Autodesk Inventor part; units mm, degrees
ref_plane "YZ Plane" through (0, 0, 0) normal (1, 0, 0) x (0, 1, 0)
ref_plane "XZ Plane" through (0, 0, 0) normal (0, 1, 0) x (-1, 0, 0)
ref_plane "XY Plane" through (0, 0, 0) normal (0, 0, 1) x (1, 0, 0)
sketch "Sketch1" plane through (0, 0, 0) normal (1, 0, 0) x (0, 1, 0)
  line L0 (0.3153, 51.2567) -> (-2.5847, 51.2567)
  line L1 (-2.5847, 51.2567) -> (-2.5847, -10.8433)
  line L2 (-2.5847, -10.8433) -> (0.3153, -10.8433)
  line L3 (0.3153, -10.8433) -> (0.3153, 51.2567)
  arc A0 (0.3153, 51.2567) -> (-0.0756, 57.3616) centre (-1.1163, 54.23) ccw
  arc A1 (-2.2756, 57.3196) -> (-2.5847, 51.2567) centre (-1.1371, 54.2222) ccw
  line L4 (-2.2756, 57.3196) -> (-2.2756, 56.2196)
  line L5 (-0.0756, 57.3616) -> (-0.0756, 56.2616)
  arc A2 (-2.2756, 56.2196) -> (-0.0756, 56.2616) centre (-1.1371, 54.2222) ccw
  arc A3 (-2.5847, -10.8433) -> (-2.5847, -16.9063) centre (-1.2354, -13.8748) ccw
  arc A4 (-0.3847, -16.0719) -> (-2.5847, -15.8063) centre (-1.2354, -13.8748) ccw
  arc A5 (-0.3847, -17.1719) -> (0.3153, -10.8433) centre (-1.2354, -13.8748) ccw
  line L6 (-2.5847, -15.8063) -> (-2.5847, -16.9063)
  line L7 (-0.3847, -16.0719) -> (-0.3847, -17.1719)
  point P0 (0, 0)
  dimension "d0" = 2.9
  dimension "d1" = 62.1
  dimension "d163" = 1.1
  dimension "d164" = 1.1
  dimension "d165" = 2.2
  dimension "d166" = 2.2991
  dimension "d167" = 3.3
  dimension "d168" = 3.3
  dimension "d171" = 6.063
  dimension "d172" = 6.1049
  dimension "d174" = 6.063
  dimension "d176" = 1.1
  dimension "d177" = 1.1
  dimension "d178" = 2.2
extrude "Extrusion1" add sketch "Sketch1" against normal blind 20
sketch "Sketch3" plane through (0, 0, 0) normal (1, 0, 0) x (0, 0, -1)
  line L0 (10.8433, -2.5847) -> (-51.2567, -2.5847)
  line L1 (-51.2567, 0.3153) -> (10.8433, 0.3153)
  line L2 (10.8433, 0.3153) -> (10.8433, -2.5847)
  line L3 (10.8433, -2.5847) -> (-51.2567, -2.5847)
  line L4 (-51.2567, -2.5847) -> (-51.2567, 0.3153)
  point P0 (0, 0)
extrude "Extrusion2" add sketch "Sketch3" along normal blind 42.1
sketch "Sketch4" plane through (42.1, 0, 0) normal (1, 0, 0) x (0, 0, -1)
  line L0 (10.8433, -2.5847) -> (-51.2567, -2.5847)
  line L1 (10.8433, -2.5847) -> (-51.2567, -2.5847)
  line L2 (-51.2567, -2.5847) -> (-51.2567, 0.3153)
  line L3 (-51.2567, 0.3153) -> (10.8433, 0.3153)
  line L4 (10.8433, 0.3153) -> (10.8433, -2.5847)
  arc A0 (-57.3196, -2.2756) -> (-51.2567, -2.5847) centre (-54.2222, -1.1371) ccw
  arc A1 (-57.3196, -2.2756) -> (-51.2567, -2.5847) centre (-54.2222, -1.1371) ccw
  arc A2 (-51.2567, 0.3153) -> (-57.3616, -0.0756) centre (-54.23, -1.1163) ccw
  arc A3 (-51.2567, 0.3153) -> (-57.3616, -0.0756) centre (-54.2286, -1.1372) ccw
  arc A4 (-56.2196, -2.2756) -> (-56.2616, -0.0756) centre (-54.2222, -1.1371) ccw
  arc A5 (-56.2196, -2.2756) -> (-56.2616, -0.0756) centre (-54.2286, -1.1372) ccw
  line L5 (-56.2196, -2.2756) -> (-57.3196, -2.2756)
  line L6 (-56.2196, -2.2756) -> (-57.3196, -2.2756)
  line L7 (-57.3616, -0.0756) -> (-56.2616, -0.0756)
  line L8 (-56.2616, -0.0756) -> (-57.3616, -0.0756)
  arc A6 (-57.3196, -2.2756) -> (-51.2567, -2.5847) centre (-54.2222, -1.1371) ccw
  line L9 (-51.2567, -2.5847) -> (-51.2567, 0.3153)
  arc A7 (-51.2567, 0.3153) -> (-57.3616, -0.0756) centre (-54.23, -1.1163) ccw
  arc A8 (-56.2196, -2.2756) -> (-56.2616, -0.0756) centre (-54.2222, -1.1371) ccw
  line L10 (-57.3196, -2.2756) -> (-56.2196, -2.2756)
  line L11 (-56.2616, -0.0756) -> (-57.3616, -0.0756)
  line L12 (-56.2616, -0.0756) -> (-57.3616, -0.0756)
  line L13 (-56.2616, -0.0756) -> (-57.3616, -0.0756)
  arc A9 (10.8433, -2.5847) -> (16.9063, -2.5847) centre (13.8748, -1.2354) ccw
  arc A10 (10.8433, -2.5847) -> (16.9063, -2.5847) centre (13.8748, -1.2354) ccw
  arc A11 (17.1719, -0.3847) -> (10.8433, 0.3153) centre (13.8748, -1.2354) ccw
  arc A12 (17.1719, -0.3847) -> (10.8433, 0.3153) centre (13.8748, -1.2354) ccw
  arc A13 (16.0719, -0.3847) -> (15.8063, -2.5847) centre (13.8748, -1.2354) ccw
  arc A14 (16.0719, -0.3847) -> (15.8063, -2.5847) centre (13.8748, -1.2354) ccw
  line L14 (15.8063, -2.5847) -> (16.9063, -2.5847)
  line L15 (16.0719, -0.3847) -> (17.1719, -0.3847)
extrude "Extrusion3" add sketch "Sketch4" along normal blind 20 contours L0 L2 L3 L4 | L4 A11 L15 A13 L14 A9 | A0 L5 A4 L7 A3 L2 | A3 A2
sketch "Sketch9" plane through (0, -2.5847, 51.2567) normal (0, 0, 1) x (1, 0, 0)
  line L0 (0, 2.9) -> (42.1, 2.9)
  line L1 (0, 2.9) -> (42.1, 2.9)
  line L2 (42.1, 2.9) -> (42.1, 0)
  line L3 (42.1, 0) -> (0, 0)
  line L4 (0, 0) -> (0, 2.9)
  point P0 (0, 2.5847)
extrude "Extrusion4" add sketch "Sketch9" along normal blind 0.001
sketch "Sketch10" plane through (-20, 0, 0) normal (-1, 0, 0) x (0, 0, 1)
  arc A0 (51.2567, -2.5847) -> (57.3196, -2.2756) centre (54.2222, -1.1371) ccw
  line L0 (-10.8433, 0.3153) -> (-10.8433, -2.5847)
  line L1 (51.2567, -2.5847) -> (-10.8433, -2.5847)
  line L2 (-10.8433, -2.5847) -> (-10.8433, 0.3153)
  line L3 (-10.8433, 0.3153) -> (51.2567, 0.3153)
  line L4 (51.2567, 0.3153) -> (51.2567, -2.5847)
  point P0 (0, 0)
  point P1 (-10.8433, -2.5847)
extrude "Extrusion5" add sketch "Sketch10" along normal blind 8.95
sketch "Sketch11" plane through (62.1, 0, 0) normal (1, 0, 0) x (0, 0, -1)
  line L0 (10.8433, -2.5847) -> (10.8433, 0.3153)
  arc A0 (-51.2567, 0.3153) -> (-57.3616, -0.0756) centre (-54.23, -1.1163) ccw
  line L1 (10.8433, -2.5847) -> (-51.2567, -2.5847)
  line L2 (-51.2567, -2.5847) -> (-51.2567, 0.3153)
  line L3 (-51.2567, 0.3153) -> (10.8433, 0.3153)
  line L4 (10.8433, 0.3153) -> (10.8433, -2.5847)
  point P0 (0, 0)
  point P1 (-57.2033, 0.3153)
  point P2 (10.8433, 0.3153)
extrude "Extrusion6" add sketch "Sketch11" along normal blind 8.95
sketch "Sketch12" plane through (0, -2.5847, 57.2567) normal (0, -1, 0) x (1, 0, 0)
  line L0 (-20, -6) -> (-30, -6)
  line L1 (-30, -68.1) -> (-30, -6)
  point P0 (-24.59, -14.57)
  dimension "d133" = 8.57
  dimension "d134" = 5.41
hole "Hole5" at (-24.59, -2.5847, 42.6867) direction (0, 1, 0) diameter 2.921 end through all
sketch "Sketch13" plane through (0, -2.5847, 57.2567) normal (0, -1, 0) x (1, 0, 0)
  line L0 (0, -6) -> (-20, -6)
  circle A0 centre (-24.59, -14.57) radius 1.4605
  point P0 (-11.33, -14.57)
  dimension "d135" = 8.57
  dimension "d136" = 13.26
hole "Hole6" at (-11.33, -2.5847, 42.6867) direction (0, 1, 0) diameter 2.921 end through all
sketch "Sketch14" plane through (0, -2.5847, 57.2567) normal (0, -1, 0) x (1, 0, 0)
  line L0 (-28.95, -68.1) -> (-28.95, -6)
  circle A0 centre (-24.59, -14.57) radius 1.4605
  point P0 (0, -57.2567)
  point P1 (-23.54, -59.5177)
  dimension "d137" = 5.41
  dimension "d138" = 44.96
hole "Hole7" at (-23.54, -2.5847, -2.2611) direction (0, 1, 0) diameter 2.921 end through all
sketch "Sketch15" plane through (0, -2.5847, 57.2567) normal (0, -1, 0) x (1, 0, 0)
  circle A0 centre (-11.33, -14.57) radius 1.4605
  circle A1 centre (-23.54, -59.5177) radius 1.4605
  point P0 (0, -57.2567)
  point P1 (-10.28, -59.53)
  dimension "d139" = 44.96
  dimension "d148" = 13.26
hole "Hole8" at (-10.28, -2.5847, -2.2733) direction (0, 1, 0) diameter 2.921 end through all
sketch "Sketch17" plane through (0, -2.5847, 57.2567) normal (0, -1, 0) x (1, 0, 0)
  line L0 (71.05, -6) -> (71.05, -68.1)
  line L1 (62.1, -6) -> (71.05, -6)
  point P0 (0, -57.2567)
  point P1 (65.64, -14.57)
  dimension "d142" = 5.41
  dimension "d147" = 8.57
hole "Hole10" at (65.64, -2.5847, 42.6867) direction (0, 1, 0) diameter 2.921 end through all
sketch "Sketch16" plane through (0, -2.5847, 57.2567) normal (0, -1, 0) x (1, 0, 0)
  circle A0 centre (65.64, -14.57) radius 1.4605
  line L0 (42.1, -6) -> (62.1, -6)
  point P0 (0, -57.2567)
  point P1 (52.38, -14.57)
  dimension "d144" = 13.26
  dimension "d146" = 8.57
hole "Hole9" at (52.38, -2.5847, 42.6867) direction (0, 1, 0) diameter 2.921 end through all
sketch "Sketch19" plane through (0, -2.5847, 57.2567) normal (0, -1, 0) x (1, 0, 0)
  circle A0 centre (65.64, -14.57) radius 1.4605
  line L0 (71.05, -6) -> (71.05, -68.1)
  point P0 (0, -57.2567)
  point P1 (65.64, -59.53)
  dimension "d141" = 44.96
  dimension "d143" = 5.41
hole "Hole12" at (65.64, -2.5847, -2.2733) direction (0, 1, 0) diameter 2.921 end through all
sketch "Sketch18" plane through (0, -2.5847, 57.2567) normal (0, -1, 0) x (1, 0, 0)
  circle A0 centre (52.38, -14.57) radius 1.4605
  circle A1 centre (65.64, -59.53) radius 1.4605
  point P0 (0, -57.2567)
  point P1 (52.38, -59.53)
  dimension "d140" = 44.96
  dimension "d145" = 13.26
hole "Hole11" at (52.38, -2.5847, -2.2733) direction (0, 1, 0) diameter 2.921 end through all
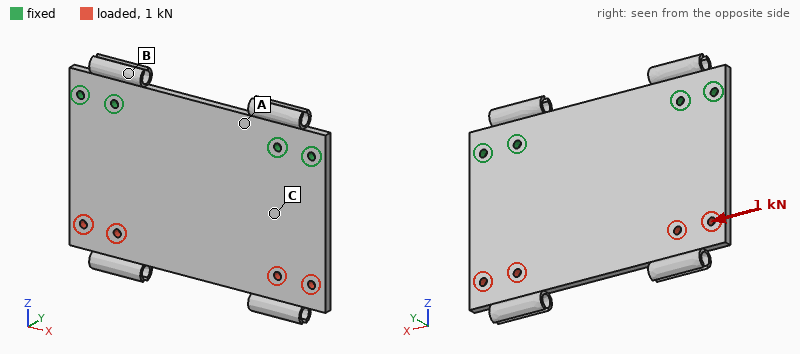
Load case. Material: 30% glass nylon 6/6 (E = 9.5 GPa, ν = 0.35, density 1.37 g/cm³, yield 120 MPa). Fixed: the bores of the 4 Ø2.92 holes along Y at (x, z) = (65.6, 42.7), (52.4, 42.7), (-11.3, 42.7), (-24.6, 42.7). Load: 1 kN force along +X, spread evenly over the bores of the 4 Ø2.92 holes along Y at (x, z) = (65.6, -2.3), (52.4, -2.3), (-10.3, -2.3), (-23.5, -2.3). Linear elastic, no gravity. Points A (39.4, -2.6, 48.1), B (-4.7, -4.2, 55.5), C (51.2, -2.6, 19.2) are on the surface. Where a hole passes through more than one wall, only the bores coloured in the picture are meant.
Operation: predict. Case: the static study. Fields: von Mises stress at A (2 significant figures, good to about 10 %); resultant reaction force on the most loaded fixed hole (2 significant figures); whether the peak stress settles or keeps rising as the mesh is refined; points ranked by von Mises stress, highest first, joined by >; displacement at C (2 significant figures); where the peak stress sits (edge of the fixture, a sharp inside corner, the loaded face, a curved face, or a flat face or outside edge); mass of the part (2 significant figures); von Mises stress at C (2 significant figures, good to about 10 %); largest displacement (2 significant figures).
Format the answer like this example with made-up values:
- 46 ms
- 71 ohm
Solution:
- 3.4 MPa
- 420 N
- keeps rising
- C > A > B
- 38 µm
- edge of the fixture
- 26 g
- 6.5 MPa
- 93 µm
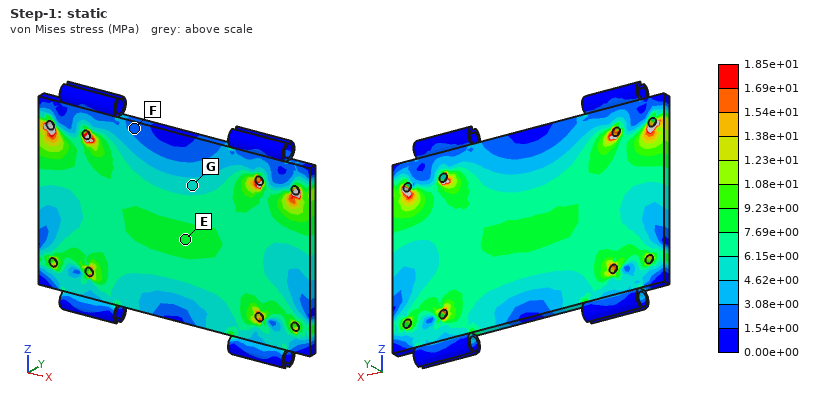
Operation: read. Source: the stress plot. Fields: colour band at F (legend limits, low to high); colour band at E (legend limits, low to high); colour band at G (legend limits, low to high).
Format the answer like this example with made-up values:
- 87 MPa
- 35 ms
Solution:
- 1.54e+00 to 3.08e+00 MPa
- 7.69e+00 to 9.23e+00 MPa
- 4.62e+00 to 6.15e+00 MPa
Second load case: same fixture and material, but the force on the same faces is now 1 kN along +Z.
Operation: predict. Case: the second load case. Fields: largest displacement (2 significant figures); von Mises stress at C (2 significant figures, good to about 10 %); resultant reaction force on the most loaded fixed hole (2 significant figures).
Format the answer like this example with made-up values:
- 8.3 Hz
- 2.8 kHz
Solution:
- 37 µm
- 4.6 MPa
- 300 N
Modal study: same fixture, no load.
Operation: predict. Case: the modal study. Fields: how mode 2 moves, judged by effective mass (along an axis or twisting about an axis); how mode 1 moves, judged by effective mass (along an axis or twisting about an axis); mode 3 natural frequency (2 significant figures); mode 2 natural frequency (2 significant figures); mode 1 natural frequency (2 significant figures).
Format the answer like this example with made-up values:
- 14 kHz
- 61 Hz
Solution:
- twisting about Z
- along Y
- 1300 Hz
- 640 Hz
- 350 Hz
